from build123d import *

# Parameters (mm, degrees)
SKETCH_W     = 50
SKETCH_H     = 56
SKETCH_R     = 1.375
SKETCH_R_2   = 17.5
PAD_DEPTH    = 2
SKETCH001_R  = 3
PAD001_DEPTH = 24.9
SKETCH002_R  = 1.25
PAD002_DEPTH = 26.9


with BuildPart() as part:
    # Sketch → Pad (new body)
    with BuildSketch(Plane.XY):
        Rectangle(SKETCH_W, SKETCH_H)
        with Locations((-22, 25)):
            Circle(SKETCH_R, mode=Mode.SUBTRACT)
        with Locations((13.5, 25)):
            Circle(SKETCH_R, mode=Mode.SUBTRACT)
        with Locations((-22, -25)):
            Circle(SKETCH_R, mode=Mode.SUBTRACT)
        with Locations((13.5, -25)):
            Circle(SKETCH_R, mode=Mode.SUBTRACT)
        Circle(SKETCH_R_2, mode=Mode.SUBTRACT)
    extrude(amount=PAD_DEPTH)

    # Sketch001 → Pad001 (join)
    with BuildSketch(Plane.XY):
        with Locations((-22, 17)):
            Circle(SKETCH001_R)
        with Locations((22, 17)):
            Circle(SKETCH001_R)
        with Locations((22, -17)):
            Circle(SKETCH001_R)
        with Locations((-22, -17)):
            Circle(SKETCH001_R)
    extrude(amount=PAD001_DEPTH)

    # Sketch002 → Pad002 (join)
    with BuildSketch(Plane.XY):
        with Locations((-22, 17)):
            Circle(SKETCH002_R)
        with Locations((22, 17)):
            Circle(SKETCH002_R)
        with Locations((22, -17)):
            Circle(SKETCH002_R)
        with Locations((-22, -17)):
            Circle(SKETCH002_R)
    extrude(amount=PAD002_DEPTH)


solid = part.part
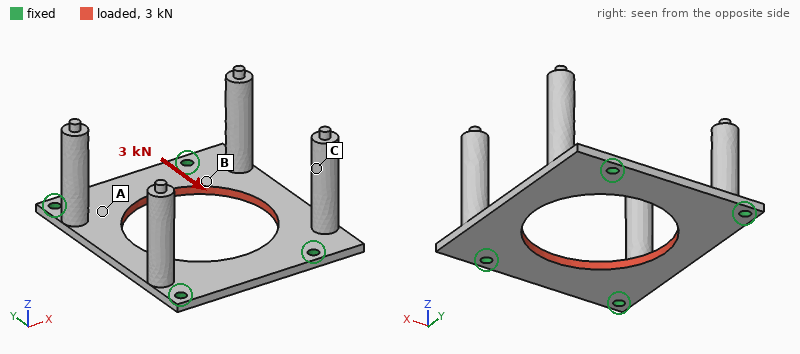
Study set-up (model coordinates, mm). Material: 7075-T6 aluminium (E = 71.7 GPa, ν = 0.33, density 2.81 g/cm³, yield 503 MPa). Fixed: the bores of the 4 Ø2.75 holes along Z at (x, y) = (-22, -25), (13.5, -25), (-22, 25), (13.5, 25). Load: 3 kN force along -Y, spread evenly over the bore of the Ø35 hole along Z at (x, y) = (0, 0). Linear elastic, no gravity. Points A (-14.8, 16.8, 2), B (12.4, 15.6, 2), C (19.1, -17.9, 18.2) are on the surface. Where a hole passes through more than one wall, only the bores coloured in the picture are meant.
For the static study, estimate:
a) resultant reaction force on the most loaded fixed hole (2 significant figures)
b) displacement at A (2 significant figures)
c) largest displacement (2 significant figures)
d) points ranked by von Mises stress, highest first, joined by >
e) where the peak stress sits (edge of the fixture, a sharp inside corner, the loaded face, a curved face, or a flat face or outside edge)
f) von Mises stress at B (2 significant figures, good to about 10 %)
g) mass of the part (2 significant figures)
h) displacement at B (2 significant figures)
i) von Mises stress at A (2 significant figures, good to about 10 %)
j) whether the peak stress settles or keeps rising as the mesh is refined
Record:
870 N
8.2 µm
14 µm
B > A > C
edge of the fixture
32 MPa
18 g
5.2 µm
17 MPa
keeps rising
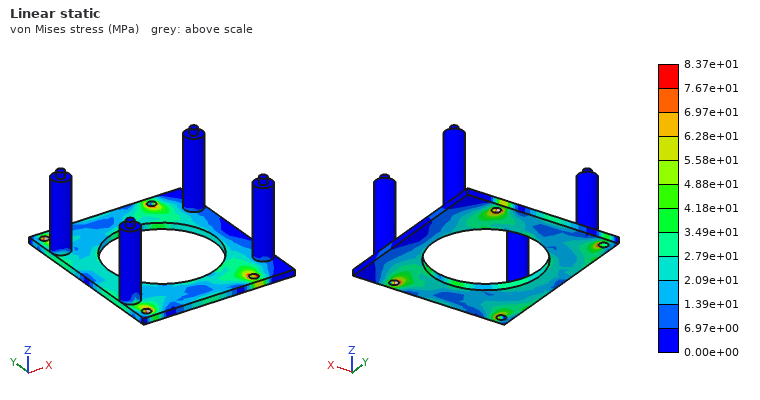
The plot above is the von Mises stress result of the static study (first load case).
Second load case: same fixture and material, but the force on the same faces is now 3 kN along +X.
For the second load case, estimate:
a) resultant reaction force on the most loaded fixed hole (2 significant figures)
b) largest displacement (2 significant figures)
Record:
900 N
31 µm
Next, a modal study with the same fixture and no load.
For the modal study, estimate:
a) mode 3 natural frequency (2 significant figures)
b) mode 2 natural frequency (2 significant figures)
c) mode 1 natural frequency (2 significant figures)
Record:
2500 Hz
2300 Hz
1900 Hz
